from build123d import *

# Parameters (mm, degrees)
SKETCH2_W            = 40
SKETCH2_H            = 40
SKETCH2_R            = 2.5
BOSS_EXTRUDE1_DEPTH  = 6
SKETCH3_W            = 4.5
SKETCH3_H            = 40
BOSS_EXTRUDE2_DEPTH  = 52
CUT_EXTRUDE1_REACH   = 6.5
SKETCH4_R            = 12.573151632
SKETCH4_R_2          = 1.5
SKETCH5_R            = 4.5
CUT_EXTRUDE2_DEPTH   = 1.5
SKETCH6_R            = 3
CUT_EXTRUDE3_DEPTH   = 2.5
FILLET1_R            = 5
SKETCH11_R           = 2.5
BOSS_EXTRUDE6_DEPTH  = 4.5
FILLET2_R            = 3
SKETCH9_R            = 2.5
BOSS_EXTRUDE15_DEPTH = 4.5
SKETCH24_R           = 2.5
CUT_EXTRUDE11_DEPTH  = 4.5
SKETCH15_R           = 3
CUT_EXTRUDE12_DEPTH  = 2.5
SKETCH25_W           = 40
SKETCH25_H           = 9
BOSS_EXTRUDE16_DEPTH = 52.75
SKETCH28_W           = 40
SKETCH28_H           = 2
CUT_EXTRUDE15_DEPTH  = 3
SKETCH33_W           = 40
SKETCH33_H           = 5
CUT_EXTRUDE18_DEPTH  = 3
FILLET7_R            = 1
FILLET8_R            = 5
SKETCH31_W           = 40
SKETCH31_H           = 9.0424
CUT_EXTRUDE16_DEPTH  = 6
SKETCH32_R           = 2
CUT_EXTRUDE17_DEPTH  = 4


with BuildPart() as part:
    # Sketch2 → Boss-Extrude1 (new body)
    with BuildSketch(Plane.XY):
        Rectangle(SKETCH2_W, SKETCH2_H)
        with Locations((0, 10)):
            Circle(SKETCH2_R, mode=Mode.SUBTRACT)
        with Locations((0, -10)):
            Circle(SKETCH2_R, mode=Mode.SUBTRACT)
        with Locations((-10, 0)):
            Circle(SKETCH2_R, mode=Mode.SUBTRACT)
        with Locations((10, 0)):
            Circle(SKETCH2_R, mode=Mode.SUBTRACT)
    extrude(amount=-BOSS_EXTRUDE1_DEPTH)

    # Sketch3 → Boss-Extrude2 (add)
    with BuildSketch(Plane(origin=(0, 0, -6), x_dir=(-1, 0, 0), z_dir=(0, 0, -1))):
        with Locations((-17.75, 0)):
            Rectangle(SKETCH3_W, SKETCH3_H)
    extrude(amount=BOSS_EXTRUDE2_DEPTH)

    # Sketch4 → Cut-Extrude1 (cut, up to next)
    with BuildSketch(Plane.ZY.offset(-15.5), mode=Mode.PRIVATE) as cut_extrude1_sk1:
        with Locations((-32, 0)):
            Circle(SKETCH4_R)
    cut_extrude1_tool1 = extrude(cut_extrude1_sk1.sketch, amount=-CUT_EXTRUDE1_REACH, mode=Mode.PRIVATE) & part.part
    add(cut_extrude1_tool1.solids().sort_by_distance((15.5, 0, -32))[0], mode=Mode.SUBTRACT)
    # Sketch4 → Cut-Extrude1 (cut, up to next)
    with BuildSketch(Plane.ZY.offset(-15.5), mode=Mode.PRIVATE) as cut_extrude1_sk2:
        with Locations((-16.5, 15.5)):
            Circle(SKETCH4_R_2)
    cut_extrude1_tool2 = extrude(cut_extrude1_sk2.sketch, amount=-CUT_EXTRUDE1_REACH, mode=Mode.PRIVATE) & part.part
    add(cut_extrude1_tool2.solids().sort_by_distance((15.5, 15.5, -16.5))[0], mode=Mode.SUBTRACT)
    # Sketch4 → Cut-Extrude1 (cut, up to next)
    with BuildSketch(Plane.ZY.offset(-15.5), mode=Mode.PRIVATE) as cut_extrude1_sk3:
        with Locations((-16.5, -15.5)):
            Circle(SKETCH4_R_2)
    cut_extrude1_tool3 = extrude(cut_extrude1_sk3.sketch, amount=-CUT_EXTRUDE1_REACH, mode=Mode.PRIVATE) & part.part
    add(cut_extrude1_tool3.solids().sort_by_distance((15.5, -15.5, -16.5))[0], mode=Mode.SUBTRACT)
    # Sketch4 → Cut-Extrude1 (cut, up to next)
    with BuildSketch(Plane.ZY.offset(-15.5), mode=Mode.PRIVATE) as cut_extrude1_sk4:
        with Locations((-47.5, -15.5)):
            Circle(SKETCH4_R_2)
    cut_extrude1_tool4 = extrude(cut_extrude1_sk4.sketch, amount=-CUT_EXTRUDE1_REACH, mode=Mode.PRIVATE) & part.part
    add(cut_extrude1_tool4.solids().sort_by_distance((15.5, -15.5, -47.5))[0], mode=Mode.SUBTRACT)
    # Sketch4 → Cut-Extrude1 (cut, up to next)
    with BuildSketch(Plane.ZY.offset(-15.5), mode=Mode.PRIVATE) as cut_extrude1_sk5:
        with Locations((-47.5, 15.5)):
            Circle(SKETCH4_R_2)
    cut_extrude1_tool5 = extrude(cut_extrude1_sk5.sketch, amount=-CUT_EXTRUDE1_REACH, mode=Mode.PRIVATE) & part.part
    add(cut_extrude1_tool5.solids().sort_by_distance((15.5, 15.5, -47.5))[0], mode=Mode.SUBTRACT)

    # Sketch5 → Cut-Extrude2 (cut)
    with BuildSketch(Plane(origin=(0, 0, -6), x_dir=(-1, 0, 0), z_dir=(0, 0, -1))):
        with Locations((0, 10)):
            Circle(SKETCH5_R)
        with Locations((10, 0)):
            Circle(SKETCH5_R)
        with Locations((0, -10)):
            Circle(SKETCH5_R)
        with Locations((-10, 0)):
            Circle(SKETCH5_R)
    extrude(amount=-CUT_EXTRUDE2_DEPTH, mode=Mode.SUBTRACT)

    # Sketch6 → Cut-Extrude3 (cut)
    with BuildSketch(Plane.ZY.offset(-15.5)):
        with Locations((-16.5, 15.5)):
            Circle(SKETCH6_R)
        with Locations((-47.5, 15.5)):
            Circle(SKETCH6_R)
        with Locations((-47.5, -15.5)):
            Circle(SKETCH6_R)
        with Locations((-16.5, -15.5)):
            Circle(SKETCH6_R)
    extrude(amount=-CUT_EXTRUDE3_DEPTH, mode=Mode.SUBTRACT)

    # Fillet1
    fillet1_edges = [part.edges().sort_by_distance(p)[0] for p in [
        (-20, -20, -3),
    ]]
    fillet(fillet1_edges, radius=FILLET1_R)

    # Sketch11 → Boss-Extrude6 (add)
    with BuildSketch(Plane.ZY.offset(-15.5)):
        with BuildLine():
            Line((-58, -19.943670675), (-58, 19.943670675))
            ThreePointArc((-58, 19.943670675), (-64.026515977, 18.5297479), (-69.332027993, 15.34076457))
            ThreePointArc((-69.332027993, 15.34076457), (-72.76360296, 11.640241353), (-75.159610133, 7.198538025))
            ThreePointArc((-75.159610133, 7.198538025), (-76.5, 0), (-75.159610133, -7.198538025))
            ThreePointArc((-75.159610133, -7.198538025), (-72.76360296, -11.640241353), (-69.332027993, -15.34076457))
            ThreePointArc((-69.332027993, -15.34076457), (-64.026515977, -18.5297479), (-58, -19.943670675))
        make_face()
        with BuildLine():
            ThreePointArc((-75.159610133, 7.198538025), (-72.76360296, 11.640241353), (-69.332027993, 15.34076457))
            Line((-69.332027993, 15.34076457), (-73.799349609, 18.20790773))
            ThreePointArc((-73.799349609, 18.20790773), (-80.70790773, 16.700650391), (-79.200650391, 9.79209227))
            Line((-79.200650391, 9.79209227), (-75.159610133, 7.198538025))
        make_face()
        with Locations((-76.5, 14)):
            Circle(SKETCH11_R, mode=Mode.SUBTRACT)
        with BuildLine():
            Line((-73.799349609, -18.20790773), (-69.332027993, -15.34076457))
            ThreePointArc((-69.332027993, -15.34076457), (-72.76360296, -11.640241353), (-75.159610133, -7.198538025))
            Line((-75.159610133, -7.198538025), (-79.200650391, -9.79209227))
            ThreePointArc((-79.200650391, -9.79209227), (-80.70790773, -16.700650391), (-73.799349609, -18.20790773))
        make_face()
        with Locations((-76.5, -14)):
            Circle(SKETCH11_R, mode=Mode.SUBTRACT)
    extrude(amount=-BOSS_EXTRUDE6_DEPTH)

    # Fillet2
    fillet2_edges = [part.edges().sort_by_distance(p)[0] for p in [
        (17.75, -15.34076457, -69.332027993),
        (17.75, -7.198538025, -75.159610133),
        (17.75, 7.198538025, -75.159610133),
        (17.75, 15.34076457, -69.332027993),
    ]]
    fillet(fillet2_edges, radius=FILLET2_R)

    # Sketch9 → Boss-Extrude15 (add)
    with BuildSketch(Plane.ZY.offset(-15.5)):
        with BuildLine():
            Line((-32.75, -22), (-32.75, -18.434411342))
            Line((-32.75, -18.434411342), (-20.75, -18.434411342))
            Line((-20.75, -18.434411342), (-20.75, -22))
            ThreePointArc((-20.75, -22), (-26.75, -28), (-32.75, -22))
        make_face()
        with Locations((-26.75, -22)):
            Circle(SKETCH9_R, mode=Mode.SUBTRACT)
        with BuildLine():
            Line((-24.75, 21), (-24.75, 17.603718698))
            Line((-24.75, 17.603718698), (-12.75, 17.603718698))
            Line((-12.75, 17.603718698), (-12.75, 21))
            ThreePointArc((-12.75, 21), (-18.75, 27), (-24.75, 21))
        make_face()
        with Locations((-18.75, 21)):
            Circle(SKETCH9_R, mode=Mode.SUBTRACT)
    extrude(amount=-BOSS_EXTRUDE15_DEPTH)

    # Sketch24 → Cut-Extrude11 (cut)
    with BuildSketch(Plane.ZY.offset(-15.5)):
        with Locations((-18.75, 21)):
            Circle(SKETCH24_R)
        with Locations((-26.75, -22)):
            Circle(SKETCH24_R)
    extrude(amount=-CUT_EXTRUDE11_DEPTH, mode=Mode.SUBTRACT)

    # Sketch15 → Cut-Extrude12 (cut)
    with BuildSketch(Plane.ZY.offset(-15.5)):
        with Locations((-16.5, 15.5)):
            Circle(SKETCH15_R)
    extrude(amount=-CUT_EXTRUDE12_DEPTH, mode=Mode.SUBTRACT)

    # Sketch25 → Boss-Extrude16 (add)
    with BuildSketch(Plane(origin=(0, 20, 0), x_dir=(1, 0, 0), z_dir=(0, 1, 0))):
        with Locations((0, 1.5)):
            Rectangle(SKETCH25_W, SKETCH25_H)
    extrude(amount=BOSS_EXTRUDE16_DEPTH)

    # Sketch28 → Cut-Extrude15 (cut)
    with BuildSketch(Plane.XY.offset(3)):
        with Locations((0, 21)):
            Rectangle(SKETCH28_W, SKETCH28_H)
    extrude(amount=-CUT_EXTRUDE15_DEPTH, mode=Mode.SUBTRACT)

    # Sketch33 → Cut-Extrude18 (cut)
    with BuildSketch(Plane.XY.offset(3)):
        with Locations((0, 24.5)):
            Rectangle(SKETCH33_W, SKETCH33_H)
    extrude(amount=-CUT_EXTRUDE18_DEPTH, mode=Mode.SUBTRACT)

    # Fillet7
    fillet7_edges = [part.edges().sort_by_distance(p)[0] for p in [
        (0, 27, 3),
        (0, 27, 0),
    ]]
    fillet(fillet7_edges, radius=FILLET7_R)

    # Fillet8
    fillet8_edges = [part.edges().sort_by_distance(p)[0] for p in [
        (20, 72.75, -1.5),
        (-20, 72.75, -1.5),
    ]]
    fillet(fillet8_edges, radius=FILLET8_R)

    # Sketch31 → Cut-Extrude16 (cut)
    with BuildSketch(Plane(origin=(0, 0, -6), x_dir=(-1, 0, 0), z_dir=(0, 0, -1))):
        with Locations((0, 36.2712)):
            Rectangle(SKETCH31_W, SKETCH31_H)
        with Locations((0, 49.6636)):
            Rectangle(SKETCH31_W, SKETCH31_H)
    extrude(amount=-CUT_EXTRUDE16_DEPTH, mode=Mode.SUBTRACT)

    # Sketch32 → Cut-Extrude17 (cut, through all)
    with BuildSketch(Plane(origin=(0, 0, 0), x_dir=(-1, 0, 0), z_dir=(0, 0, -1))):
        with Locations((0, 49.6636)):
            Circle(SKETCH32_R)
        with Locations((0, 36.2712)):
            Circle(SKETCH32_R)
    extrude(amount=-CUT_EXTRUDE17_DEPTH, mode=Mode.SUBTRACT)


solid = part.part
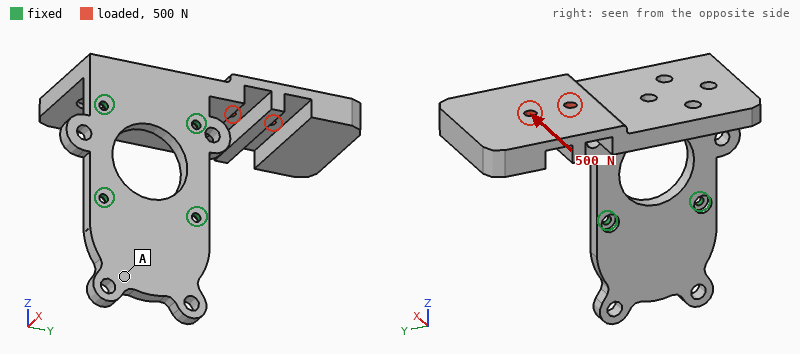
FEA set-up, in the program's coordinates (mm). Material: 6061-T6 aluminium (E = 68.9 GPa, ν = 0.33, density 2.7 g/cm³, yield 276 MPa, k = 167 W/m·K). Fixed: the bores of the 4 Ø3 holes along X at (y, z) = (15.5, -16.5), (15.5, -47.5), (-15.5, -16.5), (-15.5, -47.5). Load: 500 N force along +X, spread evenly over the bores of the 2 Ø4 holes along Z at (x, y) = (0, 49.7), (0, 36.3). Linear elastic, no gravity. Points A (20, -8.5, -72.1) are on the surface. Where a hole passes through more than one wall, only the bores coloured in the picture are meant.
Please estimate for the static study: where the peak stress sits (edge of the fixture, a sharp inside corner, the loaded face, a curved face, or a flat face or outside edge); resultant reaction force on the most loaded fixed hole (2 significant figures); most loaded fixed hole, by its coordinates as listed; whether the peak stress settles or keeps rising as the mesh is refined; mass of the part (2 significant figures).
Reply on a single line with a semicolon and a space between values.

edge of the fixture; 1.1 kN; (15.5, -16.5); keeps rising; 89 g
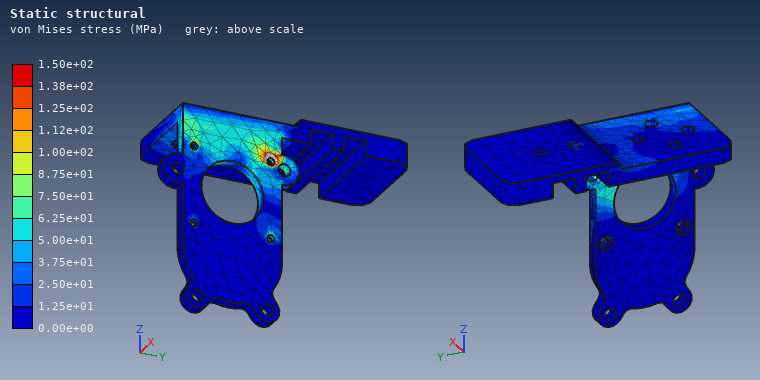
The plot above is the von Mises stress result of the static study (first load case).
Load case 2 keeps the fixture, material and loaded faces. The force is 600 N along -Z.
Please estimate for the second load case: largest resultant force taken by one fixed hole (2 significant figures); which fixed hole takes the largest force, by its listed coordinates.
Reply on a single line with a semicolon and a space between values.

780 N; (-15.5, -16.5)
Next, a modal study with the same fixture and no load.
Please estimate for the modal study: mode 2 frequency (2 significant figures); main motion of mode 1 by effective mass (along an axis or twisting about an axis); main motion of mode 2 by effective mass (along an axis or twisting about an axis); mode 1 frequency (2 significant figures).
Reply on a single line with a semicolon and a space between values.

970 Hz; along Z; along X; 560 Hz
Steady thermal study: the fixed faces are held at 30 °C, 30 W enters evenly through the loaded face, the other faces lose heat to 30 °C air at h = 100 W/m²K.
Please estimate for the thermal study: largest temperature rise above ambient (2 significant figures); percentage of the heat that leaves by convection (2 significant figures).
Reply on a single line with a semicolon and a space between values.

34 K; 65 %
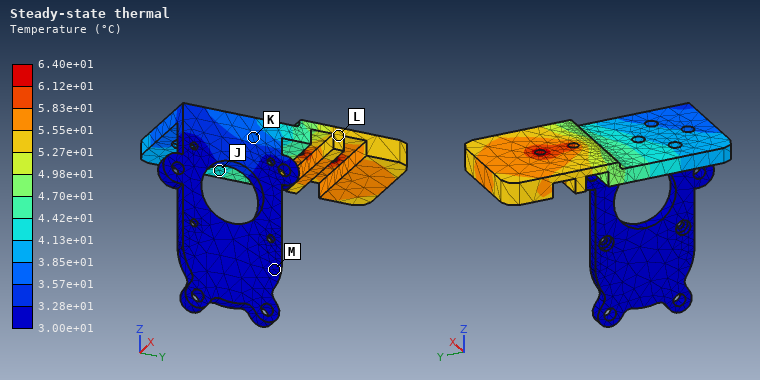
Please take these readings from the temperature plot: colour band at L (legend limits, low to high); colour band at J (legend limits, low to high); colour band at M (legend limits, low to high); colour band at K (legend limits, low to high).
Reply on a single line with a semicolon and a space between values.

5.27e+01 to 5.55e+01 °C; 4.13e+01 to 4.42e+01 °C; 3.00e+01 to 3.28e+01 °C; 3.57e+01 to 3.85e+01 °C
